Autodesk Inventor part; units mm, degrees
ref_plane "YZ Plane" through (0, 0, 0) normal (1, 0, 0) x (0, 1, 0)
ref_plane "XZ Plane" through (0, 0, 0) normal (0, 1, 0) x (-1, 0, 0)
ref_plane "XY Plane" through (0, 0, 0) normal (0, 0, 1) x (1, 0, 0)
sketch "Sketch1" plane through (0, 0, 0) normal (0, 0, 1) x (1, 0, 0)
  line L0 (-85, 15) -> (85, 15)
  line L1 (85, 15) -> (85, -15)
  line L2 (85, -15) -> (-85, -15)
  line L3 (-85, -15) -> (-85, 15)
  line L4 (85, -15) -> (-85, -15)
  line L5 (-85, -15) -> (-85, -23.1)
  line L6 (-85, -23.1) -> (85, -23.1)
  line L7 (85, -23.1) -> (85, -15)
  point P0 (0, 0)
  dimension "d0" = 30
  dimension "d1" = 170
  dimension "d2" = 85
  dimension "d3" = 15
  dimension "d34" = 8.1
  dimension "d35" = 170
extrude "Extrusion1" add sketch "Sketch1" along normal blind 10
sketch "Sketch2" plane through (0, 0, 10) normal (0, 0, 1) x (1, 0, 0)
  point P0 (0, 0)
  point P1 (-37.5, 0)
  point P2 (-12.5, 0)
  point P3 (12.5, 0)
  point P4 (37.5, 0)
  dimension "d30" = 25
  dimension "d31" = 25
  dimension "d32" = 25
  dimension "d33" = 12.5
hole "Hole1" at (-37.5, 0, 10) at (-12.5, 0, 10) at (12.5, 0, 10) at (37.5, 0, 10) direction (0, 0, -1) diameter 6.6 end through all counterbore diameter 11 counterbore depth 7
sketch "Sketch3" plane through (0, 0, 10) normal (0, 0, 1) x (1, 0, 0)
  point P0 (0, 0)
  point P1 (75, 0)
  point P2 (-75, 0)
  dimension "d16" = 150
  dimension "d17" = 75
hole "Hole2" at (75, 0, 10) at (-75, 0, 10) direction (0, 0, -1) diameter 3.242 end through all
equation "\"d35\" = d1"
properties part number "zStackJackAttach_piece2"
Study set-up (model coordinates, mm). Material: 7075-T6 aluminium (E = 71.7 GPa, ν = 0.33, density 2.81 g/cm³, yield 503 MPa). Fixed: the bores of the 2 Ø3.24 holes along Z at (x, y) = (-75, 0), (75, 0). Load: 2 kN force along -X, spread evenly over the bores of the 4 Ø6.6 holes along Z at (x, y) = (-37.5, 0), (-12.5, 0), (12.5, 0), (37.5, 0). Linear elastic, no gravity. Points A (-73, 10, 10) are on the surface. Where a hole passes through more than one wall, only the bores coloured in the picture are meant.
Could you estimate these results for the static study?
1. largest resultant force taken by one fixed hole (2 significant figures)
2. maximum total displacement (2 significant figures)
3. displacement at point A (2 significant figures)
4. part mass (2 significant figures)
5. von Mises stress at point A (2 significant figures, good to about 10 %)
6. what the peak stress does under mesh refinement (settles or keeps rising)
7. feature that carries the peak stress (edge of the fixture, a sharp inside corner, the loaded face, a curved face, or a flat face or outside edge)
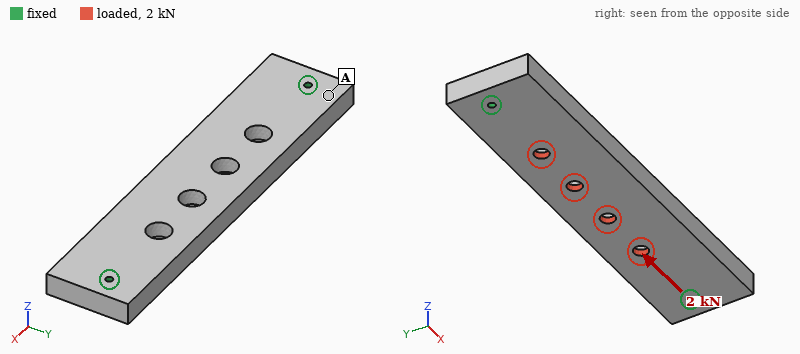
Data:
1.0 kN
4.2 µm
0.91 µm
170 g
2.1 MPa
keeps rising
edge of the fixture
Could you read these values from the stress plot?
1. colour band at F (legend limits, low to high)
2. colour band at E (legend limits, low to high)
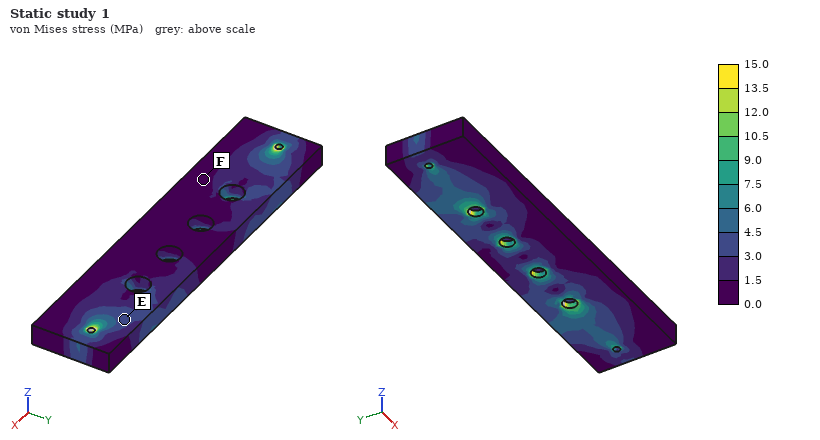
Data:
0.0 to 1.5 MPa
3.0 to 4.5 MPa
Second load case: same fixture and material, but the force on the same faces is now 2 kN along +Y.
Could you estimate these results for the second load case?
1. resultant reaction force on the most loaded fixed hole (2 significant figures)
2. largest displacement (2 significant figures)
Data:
1.2 kN
42 µm
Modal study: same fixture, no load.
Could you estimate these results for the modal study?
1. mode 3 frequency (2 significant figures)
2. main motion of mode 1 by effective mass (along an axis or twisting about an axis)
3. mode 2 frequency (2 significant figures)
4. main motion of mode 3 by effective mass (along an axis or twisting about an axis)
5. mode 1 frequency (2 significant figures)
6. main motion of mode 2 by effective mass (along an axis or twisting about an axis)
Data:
4100 Hz
along Z
3900 Hz
twisting about X
1900 Hz
along Y
